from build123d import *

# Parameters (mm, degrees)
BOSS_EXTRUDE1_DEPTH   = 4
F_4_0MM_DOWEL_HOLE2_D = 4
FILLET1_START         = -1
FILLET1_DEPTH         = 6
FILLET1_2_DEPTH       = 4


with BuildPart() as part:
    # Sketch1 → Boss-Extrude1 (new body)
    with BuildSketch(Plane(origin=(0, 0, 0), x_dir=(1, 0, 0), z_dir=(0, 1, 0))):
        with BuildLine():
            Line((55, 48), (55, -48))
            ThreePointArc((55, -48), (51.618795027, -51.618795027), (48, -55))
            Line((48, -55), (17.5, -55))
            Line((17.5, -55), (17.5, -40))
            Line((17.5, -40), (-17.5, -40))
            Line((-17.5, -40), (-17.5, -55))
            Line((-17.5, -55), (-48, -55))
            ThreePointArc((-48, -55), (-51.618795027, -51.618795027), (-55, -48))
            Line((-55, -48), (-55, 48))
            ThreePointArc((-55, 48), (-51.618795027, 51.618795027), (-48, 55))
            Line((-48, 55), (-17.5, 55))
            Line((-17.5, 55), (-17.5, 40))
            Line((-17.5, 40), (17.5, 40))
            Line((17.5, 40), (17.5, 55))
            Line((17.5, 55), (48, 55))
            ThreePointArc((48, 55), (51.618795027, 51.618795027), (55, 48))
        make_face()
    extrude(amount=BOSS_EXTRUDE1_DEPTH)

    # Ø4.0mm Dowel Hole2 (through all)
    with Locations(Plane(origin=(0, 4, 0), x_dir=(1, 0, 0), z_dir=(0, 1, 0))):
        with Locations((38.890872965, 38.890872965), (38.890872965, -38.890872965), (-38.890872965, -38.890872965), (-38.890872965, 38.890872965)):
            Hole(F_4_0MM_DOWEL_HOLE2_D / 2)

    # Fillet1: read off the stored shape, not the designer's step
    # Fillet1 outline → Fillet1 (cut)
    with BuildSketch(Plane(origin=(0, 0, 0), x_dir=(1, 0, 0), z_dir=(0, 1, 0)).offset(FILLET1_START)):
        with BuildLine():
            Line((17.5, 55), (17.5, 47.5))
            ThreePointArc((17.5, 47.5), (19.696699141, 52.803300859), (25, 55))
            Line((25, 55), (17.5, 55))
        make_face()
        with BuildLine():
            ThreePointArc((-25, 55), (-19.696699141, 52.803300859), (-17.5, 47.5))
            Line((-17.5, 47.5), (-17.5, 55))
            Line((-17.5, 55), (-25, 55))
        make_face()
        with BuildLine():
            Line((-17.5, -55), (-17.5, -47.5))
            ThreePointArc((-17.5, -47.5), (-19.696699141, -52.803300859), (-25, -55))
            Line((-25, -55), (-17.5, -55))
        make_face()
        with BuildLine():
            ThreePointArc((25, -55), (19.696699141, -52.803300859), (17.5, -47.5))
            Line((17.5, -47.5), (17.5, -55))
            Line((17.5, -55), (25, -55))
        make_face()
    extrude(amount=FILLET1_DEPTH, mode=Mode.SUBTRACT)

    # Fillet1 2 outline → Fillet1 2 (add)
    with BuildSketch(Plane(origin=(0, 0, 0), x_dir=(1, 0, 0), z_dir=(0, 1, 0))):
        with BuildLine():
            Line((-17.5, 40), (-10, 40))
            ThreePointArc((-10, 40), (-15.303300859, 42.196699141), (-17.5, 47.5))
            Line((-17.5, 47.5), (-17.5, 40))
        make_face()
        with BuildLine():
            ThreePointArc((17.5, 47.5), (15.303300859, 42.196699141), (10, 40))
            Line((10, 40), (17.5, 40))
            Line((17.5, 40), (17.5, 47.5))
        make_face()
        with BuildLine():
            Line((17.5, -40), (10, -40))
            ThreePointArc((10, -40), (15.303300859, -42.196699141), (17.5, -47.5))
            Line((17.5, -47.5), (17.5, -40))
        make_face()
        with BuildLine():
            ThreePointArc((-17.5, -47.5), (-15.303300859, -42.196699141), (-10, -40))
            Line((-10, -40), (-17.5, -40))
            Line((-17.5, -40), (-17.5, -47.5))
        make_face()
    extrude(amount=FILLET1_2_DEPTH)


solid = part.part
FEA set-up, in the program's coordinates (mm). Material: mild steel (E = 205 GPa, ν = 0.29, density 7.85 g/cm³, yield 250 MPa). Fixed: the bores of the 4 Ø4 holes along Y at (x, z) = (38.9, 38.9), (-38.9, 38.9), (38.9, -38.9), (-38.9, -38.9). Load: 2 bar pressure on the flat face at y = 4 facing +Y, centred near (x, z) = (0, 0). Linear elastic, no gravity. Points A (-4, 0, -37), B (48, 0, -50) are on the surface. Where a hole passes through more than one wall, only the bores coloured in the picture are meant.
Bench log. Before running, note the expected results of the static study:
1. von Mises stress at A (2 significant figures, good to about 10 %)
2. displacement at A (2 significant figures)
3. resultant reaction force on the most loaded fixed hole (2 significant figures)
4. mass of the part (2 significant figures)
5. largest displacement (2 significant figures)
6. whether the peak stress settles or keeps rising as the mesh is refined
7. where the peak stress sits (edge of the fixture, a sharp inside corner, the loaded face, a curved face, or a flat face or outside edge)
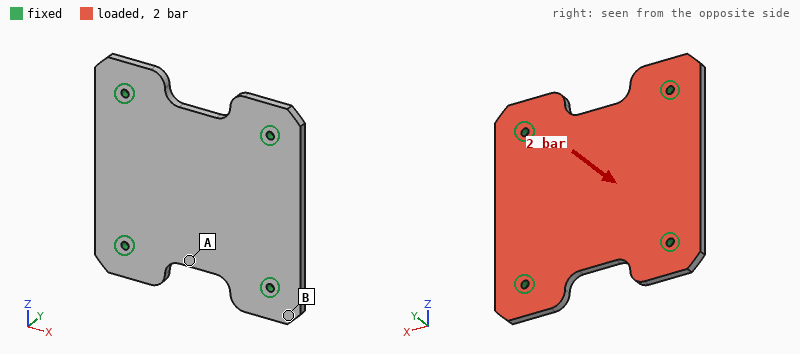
24 MPa
25 µm
550 N
340 g
45 µm
keeps rising
edge of the fixture
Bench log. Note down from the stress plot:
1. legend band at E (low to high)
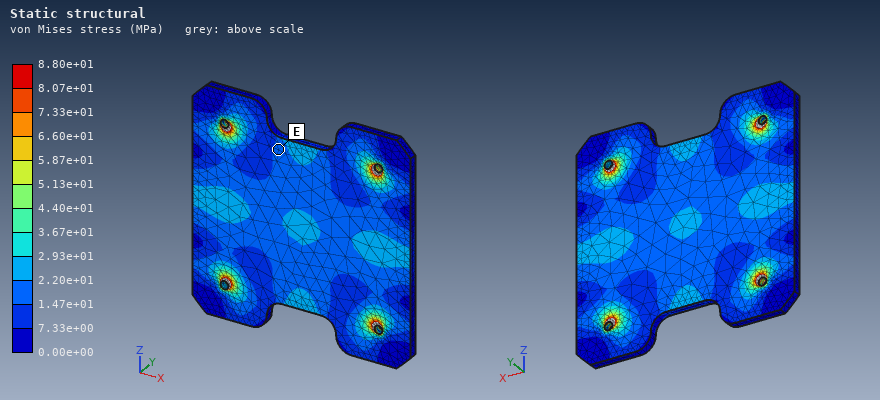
1.47e+01 to 2.20e+01 MPa
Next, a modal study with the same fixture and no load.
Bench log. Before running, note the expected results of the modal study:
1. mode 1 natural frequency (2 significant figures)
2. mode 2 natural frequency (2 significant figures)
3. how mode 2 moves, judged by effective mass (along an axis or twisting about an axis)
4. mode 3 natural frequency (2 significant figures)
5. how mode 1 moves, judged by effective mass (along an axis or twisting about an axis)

2300 Hz
3400 Hz
twisting about Z
3600 Hz
along Y
